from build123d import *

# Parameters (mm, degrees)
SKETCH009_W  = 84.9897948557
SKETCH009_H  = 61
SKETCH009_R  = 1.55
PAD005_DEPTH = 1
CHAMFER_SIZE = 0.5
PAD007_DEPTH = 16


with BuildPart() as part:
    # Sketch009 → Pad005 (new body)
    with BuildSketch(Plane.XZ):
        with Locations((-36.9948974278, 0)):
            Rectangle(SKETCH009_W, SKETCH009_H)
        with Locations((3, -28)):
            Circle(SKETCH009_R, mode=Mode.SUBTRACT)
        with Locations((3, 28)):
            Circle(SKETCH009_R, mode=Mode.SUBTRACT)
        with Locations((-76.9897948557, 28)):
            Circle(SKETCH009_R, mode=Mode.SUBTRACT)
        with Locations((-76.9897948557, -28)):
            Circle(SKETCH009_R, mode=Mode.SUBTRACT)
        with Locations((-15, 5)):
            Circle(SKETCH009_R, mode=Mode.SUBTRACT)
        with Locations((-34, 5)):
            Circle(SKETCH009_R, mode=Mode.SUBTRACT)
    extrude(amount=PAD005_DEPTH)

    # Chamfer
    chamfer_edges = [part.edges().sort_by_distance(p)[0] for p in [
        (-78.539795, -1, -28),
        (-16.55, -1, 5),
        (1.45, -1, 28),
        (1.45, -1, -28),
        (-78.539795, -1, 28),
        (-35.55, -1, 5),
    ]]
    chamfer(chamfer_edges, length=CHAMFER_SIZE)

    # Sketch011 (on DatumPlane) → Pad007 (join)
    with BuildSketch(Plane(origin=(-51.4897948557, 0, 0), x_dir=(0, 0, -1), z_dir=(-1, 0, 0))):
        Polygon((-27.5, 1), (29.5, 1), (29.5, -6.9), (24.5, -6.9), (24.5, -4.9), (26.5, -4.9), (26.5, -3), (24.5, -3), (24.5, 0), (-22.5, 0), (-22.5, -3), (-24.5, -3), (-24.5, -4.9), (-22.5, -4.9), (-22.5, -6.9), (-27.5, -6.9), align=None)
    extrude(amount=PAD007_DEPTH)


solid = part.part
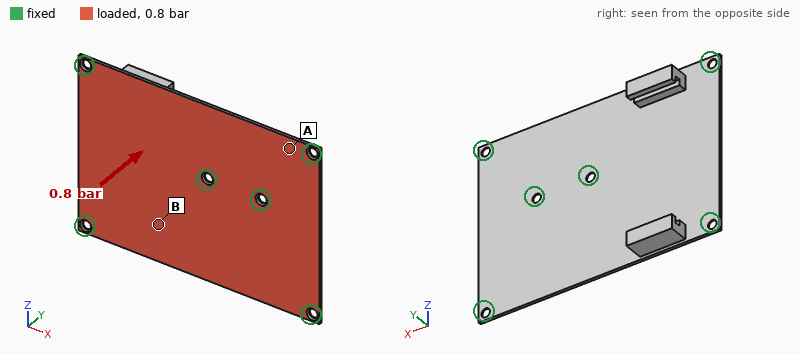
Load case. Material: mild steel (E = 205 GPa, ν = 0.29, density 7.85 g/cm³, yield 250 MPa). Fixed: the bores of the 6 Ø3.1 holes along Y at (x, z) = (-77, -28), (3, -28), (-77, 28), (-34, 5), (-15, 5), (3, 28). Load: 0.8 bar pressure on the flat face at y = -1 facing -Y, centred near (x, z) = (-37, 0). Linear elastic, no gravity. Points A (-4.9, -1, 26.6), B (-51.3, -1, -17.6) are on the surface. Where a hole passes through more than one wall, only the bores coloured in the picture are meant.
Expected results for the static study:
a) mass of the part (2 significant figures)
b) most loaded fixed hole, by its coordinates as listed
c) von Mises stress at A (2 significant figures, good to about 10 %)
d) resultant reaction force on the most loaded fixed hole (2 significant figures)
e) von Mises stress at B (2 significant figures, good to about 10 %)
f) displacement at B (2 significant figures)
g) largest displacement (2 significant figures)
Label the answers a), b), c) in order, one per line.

a) 48 g
b) (-34, 5)
c) 34 MPa
d) 170 N
e) 89 MPa
f) 0.18 mm
g) 0.28 mm
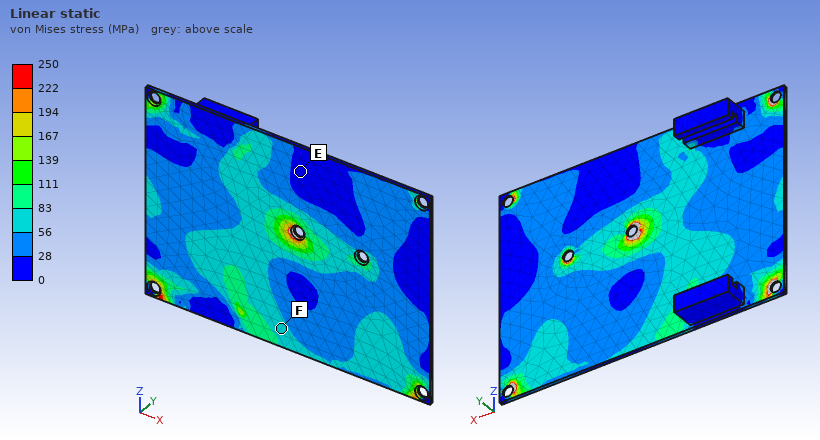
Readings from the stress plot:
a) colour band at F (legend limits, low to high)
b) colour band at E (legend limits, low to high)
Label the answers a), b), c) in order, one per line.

a) 56 to 83 MPa
b) 0 to 28 MPa
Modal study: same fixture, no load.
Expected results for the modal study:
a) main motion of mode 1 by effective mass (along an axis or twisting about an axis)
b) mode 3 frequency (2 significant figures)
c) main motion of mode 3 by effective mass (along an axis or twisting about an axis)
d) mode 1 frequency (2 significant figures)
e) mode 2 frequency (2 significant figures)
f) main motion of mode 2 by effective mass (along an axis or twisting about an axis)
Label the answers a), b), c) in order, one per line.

a) along Y
b) 1600 Hz
c) along Y
d) 1100 Hz
e) 1500 Hz
f) along Y
